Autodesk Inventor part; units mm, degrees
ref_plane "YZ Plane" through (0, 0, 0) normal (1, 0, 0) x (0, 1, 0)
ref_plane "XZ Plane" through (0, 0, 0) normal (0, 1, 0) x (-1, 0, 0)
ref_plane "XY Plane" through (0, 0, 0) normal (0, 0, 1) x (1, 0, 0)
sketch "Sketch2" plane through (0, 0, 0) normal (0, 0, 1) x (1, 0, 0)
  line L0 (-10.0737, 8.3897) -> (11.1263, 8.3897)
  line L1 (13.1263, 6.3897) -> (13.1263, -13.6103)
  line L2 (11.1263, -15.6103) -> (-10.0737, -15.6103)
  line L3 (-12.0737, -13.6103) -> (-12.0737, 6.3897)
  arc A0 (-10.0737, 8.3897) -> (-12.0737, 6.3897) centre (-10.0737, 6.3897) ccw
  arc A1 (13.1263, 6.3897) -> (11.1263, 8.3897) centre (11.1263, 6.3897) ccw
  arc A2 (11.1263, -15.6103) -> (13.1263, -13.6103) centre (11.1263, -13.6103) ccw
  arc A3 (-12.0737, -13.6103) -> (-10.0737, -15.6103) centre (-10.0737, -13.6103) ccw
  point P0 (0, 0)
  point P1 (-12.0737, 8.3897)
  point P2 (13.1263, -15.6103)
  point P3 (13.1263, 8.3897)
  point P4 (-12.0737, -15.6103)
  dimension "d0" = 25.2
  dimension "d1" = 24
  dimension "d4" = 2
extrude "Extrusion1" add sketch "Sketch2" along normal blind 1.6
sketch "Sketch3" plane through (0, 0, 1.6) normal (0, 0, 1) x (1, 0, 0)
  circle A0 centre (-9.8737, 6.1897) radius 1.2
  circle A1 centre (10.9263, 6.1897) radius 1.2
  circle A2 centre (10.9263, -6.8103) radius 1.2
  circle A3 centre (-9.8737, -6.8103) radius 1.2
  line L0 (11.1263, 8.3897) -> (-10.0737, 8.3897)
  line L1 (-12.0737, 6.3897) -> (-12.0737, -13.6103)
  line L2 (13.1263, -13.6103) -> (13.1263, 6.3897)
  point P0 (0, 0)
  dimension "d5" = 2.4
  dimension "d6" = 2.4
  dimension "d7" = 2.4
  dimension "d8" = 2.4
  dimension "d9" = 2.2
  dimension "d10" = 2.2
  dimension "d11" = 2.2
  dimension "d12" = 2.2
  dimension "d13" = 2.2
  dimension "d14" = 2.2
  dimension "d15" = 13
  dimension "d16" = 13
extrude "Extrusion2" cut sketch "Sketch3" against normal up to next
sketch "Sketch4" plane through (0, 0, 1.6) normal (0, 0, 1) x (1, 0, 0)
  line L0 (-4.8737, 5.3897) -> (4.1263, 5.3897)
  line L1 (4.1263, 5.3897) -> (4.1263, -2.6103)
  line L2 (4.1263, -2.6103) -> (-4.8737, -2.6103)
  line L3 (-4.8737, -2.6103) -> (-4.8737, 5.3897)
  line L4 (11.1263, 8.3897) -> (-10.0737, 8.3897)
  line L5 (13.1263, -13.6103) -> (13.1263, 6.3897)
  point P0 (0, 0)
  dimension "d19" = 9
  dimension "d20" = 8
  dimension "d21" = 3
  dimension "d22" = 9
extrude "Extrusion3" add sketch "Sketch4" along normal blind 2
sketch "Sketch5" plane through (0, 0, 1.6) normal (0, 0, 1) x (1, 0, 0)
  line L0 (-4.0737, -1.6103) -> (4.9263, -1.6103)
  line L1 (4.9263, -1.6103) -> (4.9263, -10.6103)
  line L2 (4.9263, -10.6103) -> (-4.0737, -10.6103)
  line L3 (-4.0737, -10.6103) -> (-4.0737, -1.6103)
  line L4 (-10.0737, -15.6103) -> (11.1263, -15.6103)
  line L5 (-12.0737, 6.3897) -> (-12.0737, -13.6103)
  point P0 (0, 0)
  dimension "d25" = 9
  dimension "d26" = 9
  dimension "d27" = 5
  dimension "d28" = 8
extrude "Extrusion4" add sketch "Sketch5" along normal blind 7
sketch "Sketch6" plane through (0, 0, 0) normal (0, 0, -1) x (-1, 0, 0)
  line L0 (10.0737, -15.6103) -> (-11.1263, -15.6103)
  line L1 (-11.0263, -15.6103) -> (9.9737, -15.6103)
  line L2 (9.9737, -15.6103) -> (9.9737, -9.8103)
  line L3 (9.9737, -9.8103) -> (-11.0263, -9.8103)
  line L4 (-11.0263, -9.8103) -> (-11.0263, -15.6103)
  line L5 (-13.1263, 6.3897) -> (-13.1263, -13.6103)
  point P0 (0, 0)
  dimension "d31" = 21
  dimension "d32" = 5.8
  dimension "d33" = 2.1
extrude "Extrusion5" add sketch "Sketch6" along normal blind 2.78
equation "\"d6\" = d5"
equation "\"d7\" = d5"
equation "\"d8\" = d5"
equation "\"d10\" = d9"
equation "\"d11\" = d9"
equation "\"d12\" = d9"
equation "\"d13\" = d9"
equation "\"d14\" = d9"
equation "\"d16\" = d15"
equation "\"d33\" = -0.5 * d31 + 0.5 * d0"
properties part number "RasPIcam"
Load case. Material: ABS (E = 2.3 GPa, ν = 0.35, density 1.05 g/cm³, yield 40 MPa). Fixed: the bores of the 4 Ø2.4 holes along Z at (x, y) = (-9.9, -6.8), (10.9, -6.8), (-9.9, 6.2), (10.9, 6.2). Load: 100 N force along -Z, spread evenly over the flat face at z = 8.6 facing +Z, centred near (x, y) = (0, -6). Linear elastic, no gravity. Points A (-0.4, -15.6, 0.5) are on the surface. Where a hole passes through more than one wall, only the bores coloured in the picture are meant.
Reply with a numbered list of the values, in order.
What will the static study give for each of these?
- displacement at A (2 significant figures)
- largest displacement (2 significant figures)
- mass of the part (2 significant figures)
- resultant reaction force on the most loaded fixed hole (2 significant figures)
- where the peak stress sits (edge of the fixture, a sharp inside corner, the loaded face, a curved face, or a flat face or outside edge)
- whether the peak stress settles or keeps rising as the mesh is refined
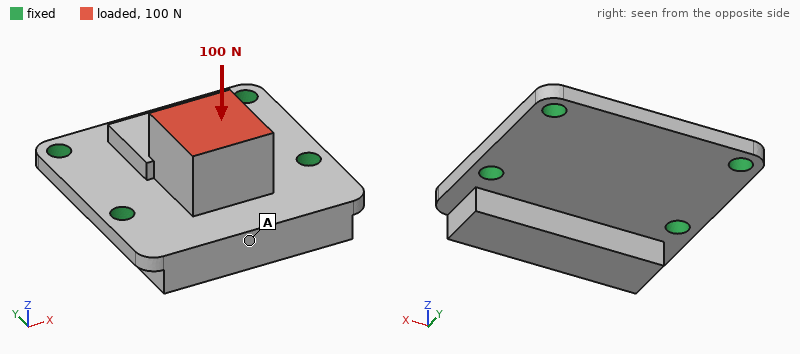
1. 0.12 mm
2. 0.12 mm
3. 2.1 g
4. 44 N
5. edge of the fixture
6. keeps rising
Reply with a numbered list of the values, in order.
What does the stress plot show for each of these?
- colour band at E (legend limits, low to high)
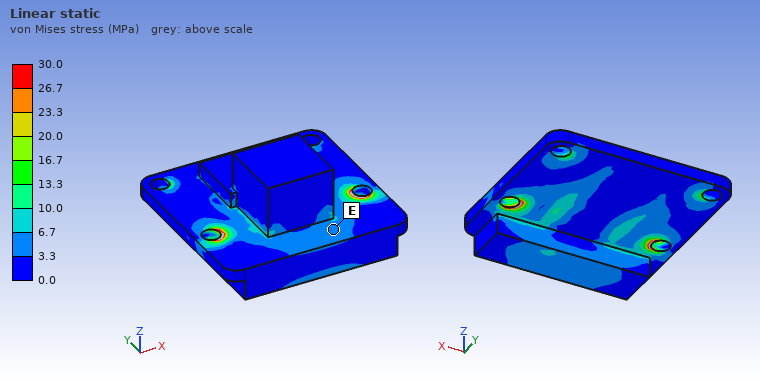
1. 3.3 to 6.7 MPa
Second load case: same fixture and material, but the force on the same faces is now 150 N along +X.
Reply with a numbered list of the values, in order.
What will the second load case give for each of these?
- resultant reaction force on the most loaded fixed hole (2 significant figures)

1. 78 N
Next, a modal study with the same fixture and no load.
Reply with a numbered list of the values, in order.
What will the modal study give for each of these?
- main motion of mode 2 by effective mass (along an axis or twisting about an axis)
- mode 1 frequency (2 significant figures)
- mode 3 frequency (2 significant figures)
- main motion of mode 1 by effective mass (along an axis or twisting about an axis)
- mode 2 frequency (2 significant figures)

1. along Z
2. 3400 Hz
3. 7700 Hz
4. along Z
5. 5200 Hz
